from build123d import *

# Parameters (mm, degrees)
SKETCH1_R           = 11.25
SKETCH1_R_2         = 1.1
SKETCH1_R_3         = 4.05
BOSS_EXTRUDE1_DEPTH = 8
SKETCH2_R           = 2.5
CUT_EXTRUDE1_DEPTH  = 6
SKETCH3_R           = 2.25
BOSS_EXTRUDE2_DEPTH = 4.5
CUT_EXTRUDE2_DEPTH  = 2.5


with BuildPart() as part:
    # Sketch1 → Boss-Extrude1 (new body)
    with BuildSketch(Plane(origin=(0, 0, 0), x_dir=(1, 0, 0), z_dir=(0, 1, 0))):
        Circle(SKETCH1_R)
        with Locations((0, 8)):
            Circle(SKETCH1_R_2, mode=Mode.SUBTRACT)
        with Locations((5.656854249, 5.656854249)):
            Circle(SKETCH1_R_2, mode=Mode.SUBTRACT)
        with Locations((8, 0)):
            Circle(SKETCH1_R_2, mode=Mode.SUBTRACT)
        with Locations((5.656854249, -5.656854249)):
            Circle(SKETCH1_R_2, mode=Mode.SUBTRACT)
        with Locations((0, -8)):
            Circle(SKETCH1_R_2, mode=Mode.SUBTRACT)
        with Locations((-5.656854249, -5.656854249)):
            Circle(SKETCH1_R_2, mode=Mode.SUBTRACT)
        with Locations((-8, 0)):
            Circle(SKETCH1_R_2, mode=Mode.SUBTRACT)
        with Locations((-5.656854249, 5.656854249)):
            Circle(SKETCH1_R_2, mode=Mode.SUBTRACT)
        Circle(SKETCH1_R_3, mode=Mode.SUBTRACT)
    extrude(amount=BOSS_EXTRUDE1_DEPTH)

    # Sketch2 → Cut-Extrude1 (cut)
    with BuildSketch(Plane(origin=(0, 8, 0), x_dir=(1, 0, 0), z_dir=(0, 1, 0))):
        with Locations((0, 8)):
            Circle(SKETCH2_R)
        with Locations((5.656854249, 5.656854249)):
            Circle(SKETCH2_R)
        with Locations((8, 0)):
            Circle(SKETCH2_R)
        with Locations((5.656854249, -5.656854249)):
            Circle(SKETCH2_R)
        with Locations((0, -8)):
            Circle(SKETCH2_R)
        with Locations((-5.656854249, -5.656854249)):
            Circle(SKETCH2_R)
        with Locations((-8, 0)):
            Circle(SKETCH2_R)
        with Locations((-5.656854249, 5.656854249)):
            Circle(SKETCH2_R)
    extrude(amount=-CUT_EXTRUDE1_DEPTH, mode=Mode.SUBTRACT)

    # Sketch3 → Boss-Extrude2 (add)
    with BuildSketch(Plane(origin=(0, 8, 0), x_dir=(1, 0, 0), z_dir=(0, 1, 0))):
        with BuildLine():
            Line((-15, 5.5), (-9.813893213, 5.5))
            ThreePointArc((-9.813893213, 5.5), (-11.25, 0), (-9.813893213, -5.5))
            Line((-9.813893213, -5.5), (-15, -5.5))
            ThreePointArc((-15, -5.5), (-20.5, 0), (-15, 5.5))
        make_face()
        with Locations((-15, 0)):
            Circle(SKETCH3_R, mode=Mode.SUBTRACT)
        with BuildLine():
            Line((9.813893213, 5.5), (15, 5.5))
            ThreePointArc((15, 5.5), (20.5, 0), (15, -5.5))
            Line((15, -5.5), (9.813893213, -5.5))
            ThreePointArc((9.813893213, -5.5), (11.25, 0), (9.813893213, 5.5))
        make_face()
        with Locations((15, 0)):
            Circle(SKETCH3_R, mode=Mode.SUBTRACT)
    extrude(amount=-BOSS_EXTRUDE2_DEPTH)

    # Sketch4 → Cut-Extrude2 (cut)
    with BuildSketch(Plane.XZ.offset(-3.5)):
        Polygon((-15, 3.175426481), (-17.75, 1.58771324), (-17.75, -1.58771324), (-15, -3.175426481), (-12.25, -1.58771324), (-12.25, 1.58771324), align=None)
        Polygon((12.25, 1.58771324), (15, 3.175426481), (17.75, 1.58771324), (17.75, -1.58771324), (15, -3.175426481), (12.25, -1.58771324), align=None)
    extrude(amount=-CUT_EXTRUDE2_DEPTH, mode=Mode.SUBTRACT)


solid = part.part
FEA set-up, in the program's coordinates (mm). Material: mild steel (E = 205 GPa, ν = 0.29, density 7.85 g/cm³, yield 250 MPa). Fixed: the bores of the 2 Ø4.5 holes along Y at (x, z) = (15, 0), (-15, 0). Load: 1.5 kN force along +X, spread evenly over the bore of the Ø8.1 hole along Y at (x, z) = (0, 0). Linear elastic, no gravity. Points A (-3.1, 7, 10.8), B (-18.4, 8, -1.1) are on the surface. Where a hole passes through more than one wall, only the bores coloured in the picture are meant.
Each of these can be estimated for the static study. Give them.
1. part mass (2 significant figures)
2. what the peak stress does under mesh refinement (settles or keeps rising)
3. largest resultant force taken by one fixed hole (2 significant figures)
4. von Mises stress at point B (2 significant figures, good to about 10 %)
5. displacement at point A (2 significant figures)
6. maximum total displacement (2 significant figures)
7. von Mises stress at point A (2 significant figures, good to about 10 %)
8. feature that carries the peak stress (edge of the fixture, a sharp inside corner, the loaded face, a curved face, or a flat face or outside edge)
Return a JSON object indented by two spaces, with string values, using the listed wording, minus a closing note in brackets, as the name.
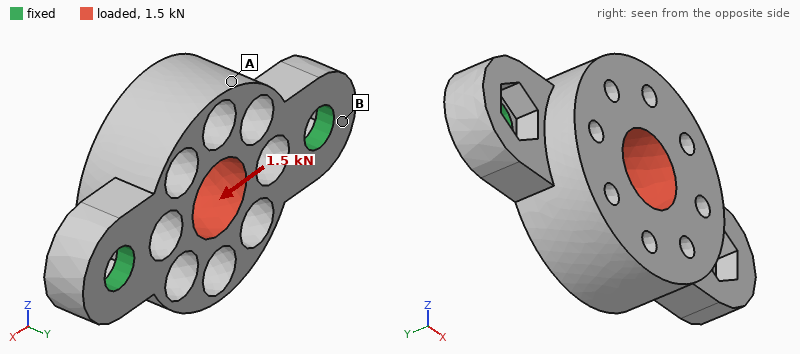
{
  "part mass": "19 g",
  "what the peak stress does under mesh refinement": "keeps rising",
  "largest resultant force taken by one fixed hole": "760 N",
  "von Mises stress at point B": "14 MPa",
  "displacement at point A": "2.0 µm",
  "maximum total displacement": "2.9 µm",
  "von Mises stress at point A": "7.6 MPa",
  "feature that carries the peak stress": "edge of the fixture"
}
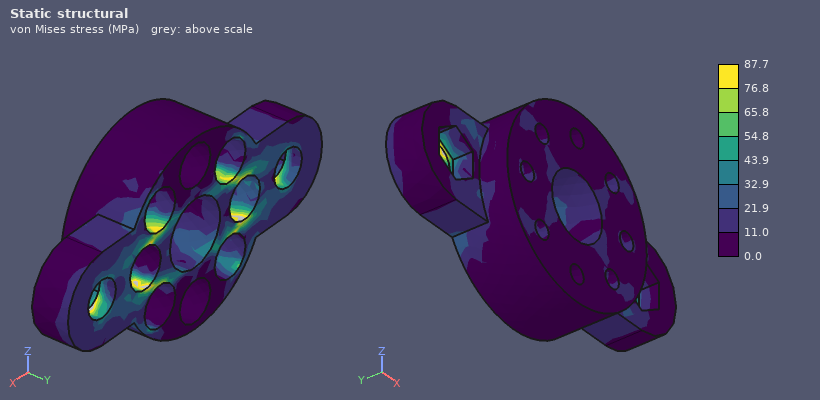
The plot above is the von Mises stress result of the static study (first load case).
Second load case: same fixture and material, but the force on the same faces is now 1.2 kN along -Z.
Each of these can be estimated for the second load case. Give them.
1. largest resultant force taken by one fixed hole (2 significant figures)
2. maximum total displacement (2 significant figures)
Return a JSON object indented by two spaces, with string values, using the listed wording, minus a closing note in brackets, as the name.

{
  "largest resultant force taken by one fixed hole": "600 N",
  "maximum total displacement": "11 µm"
}
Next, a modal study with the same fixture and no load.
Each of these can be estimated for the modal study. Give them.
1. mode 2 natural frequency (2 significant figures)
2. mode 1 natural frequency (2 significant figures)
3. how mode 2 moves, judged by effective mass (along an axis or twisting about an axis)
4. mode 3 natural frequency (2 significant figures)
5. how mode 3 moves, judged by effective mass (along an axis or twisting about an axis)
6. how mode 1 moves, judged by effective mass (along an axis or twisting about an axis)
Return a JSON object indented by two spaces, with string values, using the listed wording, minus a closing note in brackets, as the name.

{
  "mode 2 natural frequency": "21 kHz",
  "mode 1 natural frequency": "12 kHz",
  "how mode 2 moves, judged by effective mass": "along Y",
  "mode 3 natural frequency": "30 kHz",
  "how mode 3 moves, judged by effective mass": "along Z",
  "how mode 1 moves, judged by effective mass": "along Z"
}
